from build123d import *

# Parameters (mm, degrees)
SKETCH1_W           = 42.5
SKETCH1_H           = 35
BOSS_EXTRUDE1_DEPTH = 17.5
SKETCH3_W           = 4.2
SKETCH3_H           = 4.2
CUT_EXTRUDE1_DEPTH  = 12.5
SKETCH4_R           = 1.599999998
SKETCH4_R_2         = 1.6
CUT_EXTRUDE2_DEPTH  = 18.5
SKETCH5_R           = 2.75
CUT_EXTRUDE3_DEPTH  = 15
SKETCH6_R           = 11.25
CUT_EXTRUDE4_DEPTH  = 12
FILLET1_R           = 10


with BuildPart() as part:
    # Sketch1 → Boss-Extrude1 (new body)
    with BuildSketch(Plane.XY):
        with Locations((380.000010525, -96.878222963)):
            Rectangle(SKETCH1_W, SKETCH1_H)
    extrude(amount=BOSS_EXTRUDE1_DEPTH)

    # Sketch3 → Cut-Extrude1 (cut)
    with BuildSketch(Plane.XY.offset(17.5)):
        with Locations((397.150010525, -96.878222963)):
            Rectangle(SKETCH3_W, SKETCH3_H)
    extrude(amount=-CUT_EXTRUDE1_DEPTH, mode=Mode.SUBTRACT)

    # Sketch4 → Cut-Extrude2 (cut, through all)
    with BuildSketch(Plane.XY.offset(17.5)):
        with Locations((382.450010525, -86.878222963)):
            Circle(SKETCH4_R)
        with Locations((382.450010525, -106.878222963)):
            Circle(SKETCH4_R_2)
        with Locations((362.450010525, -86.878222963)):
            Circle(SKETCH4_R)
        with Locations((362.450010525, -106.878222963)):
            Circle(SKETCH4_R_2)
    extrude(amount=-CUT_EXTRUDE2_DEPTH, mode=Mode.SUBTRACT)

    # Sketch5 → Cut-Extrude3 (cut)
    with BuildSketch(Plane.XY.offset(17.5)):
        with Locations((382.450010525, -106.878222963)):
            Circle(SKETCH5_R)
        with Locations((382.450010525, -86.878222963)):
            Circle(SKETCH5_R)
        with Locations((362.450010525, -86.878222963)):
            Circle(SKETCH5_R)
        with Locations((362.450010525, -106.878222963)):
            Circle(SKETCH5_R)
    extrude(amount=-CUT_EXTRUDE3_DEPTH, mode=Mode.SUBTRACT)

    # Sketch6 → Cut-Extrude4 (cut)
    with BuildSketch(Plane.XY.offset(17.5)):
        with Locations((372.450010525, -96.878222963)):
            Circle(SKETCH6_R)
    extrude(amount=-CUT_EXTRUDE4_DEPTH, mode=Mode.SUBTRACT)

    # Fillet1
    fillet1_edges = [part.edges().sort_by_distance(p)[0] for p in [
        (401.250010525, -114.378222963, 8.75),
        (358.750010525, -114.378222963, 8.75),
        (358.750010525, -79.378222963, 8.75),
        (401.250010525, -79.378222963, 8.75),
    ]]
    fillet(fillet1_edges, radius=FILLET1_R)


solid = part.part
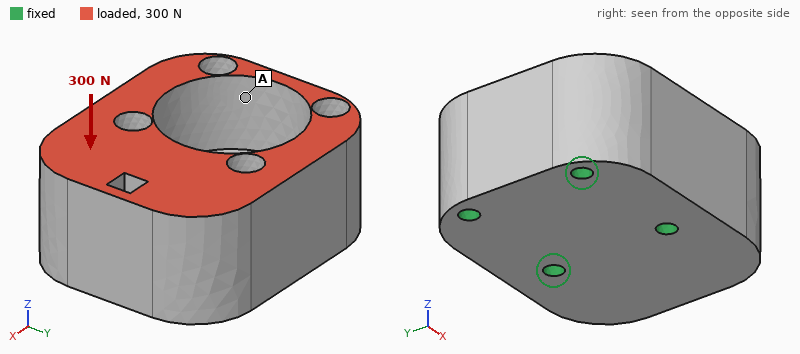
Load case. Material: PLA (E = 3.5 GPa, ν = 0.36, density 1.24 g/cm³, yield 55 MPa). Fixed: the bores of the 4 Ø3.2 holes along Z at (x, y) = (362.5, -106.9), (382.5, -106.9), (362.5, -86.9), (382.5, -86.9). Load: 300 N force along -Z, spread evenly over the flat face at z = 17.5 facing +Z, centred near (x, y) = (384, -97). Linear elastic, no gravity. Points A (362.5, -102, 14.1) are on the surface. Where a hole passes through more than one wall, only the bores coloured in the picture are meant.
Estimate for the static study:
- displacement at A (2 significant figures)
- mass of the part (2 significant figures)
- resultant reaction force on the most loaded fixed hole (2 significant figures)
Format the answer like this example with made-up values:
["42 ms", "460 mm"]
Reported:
["8.0 µm", "22 g", "160 N"]
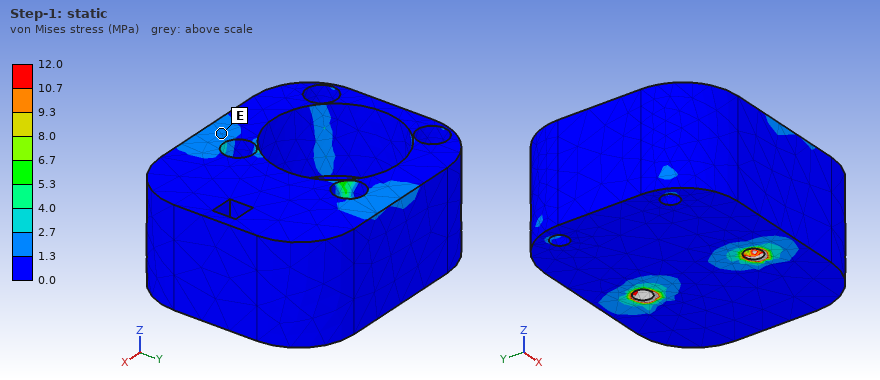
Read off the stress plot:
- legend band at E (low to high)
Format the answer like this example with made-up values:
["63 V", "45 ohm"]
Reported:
["1.3 to 2.7 MPa"]
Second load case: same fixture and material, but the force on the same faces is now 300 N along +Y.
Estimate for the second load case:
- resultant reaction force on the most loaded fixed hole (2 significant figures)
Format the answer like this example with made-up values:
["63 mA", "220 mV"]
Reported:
["210 N"]
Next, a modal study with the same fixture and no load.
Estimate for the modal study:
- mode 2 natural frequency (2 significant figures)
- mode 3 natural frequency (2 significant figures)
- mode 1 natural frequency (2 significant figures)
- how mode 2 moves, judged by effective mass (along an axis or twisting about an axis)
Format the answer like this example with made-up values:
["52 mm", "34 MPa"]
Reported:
["4200 Hz", "6200 Hz", "3200 Hz", "along Y"]
